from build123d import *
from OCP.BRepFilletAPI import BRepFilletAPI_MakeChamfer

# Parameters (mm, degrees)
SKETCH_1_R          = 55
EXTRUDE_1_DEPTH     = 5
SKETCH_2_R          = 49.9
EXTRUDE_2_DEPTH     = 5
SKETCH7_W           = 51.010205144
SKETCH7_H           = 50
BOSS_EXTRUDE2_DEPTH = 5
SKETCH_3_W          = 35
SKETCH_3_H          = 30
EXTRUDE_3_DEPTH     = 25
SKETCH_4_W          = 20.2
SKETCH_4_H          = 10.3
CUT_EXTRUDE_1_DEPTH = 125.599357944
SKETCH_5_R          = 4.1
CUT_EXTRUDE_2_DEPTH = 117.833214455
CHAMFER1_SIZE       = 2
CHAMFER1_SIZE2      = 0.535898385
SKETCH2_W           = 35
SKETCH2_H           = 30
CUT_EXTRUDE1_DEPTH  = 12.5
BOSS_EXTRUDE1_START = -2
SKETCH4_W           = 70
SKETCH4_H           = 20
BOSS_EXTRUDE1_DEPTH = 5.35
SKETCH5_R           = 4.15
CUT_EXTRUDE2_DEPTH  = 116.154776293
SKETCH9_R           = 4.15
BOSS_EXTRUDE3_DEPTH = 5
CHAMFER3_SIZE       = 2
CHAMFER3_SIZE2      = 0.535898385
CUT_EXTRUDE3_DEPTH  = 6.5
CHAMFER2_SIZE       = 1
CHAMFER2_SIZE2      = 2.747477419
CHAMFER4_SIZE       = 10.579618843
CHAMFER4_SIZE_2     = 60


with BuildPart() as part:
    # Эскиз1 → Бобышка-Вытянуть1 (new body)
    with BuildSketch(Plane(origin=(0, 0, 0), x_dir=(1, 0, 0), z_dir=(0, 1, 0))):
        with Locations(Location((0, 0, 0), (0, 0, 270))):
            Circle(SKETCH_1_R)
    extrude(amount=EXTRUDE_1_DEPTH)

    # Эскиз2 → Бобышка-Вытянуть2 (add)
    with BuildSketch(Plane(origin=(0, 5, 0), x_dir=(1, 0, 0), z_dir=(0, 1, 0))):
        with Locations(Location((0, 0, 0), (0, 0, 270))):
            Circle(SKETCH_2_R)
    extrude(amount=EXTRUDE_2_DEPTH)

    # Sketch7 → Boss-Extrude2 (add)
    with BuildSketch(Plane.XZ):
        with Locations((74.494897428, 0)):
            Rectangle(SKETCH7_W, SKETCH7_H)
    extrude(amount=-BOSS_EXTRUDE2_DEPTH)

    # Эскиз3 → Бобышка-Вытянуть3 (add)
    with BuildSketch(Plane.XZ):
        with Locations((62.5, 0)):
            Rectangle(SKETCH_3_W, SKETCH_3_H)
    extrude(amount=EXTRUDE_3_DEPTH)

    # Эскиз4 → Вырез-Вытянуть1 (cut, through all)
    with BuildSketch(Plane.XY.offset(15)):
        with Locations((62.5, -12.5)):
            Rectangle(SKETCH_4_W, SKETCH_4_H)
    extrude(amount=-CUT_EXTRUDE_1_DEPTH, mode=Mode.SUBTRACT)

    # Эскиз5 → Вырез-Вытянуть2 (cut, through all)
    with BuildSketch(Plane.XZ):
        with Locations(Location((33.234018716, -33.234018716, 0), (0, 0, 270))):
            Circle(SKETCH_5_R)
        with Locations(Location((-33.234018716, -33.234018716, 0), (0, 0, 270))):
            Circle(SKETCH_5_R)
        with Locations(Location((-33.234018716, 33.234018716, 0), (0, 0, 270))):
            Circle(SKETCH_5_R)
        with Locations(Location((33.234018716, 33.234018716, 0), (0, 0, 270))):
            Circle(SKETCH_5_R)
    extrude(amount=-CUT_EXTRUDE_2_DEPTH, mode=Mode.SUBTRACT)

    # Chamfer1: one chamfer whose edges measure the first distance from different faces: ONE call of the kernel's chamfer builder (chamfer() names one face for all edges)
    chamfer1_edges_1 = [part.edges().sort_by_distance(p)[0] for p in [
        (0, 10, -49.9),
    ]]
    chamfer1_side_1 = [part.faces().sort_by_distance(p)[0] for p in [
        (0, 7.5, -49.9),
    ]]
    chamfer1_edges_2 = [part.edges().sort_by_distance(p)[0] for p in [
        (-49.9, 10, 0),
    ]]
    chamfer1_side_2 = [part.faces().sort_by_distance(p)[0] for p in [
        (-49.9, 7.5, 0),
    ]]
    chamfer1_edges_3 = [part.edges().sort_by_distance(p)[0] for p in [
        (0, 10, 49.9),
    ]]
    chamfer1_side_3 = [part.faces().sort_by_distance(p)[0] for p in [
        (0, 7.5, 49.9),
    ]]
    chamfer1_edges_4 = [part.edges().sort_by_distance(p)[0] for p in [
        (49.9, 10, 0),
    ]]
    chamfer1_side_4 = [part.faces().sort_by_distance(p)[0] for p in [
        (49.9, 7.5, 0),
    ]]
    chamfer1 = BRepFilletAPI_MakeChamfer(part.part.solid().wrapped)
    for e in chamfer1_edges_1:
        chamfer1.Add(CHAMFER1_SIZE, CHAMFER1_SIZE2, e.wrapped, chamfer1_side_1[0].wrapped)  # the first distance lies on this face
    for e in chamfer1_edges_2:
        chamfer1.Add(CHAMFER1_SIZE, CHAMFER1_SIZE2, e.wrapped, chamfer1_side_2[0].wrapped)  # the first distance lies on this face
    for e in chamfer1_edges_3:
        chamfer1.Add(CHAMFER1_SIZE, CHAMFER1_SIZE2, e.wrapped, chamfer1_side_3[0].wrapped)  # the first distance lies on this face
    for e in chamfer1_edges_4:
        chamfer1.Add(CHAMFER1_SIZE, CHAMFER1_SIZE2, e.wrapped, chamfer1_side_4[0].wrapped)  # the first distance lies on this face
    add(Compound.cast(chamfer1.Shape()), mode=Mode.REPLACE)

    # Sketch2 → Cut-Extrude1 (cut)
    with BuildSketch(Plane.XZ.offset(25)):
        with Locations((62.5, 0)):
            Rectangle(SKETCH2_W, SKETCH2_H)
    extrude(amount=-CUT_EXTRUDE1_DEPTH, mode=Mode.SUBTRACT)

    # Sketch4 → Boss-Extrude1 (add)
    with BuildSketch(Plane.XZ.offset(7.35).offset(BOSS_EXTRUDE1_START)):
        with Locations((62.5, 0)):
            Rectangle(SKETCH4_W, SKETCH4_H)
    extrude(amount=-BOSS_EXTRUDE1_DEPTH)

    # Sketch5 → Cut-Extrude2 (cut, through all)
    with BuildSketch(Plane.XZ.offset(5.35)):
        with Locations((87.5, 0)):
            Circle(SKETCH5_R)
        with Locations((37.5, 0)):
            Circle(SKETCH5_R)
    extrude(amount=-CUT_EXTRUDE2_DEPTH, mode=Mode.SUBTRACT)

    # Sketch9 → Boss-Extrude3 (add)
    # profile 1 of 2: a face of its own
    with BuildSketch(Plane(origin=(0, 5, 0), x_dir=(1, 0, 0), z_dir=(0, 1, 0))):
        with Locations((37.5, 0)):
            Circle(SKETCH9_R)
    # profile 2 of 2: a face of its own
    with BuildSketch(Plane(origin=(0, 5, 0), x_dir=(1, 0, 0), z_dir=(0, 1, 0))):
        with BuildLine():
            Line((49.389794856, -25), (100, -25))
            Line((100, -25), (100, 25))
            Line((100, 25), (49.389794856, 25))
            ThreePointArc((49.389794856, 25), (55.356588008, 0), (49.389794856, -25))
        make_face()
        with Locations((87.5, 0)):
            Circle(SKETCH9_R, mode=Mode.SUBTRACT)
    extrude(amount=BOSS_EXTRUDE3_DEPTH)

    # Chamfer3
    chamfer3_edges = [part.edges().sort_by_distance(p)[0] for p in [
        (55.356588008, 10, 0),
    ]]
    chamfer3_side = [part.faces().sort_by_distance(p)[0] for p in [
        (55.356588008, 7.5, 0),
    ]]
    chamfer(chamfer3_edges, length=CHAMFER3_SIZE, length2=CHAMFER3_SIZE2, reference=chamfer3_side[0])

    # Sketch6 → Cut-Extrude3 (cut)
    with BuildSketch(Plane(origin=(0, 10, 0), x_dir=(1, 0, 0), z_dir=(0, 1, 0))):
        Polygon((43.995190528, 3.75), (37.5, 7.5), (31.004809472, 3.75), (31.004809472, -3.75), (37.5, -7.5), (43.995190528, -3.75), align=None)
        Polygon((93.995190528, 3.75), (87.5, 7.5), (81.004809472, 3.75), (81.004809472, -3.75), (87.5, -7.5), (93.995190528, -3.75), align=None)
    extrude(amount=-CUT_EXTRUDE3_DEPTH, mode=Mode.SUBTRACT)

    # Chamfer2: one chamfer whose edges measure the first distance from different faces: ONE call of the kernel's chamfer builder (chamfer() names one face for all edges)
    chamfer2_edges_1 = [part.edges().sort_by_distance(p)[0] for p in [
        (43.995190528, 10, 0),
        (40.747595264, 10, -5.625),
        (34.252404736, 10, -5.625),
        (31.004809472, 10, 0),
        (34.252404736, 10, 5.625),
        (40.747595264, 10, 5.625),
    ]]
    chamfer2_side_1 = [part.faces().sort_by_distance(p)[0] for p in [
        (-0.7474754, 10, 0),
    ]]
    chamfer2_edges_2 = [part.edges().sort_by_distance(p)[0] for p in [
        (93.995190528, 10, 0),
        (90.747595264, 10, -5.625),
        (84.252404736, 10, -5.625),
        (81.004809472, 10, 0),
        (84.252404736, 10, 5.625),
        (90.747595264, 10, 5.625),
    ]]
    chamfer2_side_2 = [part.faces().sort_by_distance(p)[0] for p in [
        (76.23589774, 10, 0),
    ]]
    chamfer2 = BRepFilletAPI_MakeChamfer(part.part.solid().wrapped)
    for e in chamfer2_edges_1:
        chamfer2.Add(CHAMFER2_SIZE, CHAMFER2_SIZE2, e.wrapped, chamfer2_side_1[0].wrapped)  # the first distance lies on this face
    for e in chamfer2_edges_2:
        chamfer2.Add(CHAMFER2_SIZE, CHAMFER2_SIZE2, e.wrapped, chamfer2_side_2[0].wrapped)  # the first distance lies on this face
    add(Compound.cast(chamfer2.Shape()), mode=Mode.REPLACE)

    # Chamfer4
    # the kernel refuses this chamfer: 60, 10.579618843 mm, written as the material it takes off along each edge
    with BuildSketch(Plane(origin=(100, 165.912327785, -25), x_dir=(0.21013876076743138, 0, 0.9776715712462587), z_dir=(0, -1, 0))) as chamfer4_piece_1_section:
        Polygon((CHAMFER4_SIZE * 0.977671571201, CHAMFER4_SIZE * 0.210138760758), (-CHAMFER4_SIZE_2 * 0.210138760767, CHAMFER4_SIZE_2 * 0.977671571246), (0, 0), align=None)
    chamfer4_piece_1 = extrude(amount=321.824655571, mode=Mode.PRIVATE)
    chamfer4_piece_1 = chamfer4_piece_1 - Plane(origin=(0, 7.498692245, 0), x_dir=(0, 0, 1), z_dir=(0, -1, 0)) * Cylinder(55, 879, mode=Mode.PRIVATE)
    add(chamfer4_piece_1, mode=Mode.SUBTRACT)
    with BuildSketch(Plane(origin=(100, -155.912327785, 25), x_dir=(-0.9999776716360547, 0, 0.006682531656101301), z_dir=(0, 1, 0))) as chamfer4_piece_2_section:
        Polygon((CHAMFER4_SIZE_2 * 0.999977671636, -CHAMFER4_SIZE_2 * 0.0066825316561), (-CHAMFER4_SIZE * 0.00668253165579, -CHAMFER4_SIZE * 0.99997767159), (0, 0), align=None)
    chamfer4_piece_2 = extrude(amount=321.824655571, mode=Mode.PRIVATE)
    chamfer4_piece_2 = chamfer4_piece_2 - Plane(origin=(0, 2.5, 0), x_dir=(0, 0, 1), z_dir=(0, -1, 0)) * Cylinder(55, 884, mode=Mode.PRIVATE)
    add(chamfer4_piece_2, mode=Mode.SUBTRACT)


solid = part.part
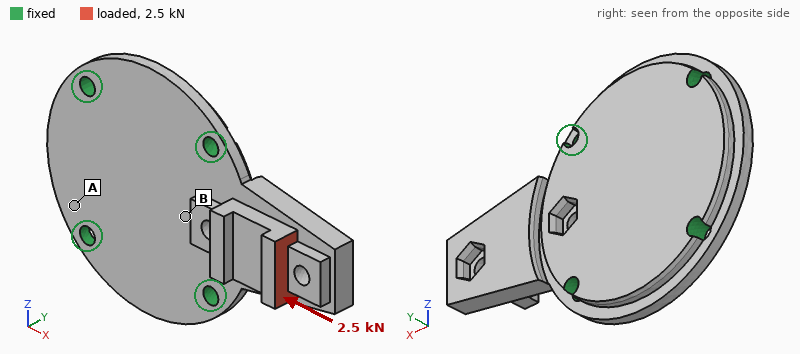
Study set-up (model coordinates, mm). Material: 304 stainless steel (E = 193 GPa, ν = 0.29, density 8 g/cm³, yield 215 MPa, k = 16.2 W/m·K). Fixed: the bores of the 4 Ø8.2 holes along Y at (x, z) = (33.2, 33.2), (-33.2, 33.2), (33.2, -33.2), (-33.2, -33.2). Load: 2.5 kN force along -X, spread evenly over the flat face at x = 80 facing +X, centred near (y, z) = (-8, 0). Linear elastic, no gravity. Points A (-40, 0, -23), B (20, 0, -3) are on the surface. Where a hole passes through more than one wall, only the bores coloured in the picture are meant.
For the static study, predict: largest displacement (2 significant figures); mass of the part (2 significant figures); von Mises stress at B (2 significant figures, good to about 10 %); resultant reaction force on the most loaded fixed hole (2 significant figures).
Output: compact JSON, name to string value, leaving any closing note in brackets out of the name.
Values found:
{"largest displacement": "59 µm", "mass of the part": "900 g", "von Mises stress at B": "16 MPa", "resultant reaction force on the most loaded fixed hole": "830 N"}
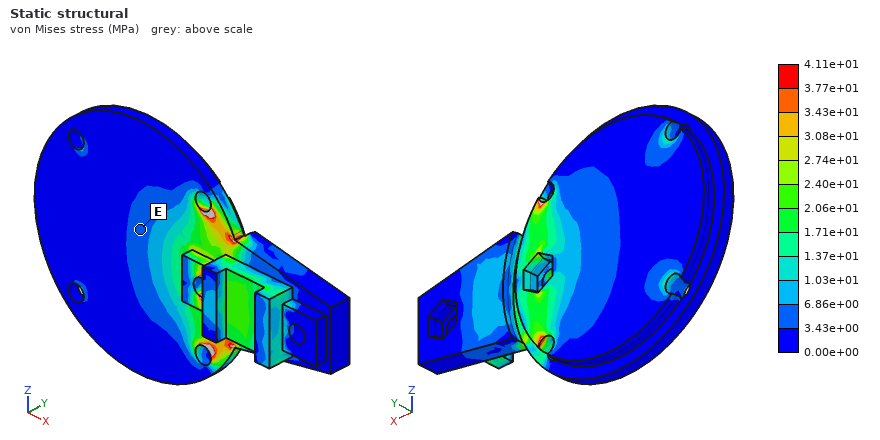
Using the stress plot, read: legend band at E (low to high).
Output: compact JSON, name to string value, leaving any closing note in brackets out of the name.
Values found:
{"legend band at E": "3.43e+00 to 6.86e+00 MPa"}
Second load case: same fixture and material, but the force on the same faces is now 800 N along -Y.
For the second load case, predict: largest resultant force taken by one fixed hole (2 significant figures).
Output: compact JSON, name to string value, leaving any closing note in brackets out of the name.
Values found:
{"largest resultant force taken by one fixed hole": "630 N"}
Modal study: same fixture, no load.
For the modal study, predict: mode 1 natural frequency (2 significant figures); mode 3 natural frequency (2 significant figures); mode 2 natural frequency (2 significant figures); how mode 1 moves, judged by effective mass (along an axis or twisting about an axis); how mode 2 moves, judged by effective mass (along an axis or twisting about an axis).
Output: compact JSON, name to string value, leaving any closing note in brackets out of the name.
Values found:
{"mode 1 natural frequency": "1600 Hz", "mode 3 natural frequency": "7500 Hz", "mode 2 natural frequency": "6500 Hz", "how mode 1 moves, judged by effective mass": "along Y", "how mode 2 moves, judged by effective mass": "along Z"}
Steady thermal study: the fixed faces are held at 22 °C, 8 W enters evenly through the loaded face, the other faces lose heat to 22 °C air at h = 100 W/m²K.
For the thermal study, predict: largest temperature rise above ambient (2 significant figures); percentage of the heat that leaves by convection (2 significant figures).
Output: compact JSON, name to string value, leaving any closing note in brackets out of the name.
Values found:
{"largest temperature rise above ambient": "26 K", "percentage of the heat that leaves by convection": "91 %"}
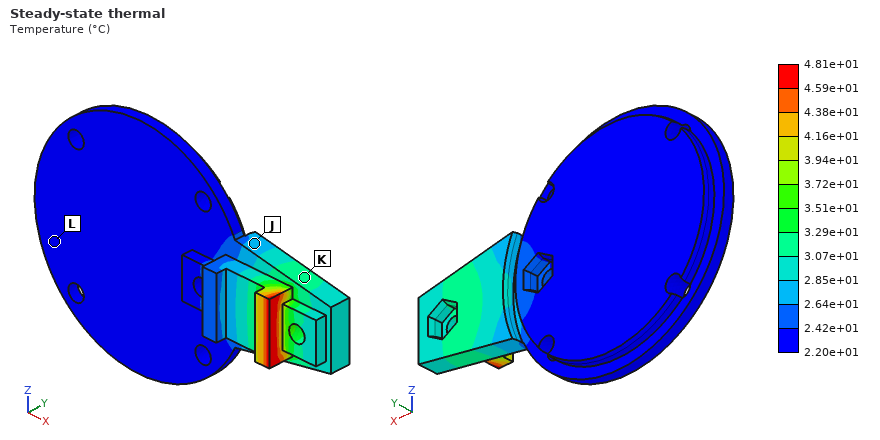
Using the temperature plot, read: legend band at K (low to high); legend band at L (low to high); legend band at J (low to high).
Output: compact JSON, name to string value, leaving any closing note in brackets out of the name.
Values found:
{"legend band at K": "3.07e+01 to 3.29e+01 °C", "legend band at L": "2.20e+01 to 2.42e+01 °C", "legend band at J": "2.64e+01 to 2.85e+01 °C"}
